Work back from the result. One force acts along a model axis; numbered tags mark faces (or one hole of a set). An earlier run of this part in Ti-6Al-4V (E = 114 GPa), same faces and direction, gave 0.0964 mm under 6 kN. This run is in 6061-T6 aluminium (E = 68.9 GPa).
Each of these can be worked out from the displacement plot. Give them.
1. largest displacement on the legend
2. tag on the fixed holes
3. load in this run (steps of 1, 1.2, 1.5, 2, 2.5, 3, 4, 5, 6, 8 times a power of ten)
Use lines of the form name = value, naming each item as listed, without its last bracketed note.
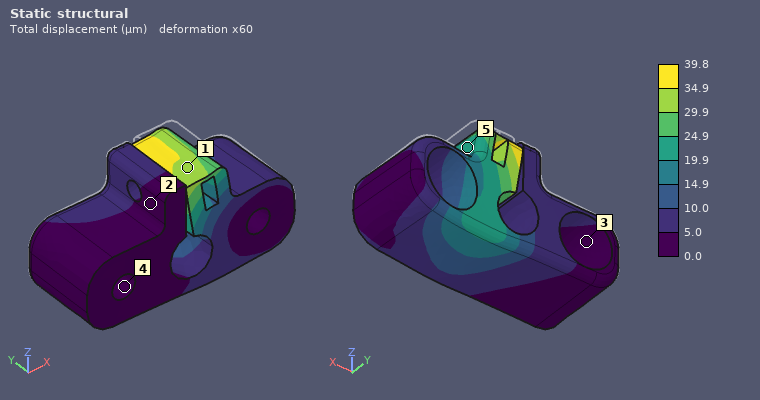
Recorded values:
largest displacement on the legend = 39.8 µm
tag on the fixed holes = 4
load in this run = 1.5 kN
